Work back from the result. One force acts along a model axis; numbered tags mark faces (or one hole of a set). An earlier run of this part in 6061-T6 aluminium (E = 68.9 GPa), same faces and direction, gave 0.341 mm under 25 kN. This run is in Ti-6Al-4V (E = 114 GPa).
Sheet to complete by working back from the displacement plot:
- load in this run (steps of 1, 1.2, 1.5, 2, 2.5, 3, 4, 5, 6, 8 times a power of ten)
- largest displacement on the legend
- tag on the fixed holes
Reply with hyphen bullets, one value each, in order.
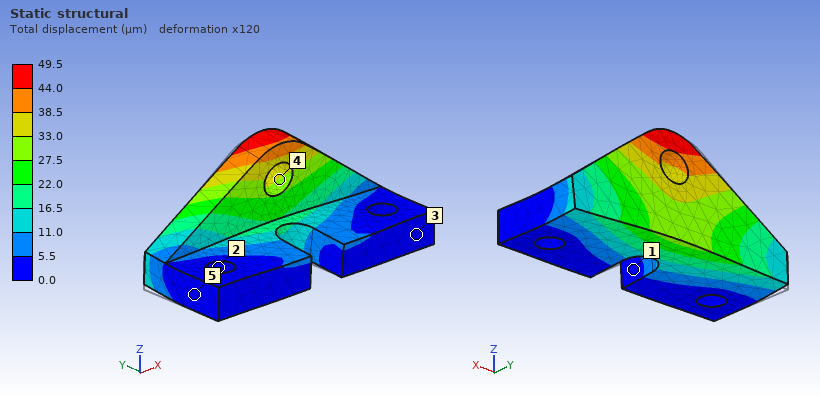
- 6 kN
- 49.5 µm
- 2
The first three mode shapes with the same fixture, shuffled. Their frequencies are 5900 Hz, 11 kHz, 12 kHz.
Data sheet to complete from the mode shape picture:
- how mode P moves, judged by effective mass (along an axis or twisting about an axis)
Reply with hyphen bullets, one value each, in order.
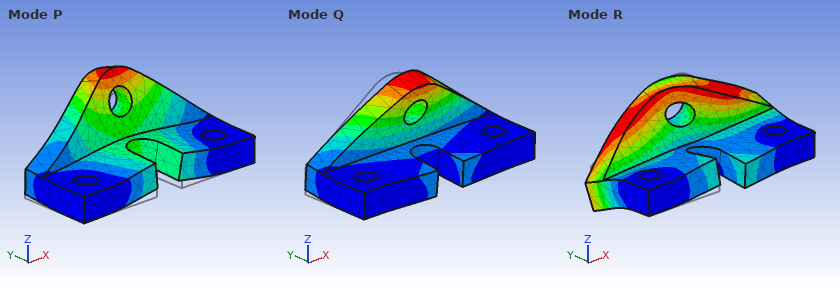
- along Z
